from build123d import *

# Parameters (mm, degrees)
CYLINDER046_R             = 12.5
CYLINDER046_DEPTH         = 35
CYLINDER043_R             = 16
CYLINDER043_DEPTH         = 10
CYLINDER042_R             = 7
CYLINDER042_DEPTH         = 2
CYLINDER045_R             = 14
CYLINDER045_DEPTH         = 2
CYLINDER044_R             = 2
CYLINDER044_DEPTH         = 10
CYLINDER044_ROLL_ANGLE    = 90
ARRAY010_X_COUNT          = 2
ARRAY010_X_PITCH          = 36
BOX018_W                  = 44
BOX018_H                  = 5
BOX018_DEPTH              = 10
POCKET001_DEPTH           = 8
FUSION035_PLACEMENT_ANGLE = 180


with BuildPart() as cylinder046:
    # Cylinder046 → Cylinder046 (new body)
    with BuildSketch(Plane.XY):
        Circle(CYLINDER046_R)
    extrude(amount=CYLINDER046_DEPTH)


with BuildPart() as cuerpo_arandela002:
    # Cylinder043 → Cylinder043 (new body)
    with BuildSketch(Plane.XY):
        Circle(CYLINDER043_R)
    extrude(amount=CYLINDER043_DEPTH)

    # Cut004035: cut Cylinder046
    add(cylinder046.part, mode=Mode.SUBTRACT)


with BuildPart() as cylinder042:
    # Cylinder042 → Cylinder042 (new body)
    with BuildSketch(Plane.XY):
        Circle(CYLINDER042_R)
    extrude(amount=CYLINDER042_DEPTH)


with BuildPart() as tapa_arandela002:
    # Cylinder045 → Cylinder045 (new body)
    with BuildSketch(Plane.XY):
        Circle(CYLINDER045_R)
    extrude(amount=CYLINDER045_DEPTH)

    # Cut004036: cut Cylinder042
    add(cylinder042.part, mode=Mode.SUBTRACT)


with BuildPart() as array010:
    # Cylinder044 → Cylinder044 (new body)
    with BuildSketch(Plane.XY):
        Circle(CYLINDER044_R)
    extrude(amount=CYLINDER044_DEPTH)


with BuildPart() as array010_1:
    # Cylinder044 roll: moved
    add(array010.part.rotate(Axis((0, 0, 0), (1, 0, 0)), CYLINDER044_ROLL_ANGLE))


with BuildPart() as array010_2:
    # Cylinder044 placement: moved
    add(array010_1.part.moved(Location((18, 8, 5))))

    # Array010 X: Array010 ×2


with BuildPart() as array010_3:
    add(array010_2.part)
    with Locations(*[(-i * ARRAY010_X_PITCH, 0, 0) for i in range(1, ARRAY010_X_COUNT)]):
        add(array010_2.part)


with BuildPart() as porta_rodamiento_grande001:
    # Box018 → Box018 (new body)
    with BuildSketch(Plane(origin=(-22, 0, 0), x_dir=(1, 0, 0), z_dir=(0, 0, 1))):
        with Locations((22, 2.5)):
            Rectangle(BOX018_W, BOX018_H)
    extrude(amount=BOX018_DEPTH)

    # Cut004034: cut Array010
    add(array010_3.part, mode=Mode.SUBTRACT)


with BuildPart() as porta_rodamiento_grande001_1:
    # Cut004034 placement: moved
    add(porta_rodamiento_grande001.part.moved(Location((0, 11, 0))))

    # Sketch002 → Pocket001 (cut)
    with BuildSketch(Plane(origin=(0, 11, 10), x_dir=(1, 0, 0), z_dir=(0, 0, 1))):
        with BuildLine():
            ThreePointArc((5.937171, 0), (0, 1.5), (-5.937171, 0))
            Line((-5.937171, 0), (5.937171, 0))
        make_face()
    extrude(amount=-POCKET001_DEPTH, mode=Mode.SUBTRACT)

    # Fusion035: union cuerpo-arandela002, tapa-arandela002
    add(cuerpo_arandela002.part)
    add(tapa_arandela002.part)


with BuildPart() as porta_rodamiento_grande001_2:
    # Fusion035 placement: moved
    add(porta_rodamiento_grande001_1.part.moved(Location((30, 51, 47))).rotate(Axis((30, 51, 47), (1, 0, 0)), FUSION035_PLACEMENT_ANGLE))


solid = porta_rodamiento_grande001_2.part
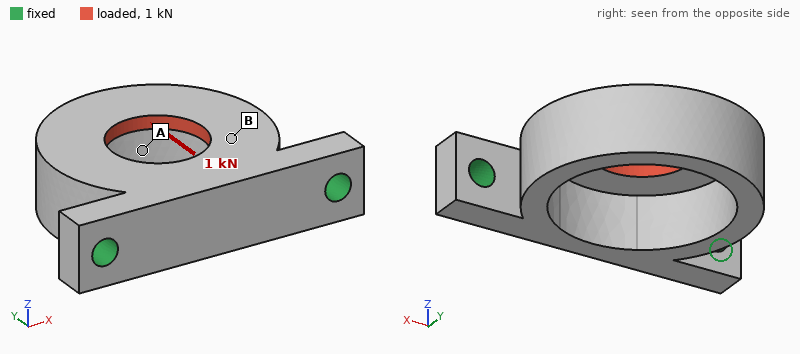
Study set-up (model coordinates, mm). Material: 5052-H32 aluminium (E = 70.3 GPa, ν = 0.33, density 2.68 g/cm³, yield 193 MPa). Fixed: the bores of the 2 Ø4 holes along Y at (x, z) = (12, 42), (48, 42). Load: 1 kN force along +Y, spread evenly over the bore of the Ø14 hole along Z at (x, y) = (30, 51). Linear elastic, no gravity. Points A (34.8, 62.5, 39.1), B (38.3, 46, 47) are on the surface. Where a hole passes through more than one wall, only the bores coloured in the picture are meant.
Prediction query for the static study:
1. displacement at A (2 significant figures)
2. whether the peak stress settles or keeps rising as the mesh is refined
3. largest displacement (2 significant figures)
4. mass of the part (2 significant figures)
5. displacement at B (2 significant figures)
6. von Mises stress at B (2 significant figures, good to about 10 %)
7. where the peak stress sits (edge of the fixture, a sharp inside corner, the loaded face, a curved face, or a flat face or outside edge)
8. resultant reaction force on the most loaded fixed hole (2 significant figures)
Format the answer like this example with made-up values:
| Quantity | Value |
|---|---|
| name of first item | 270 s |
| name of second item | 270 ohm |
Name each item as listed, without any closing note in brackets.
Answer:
| Quantity | Value |
|---|---|
| displacement at A | 49 µm |
| whether the peak stress settles or keeps rising as the mesh is refined | keeps rising |
| largest displacement | 64 µm |
| mass of the part | 14 g |
| displacement at B | 23 µm |
| von Mises stress at B | 27 MPa |
| where the peak stress sits | edge of the fixture |
| resultant reaction force on the most loaded fixed hole | 510 N |
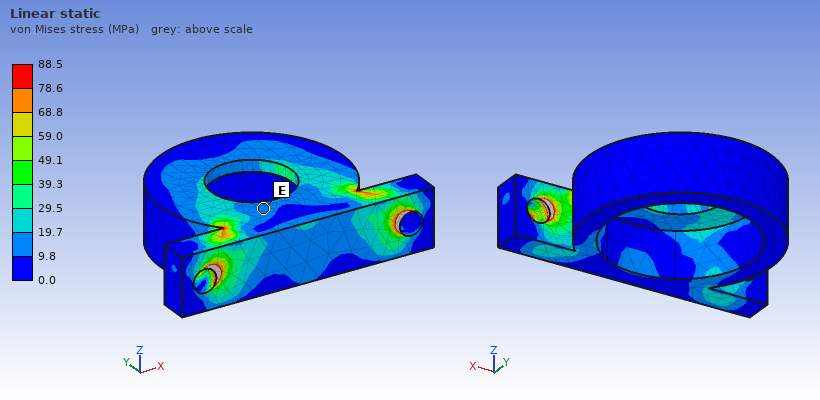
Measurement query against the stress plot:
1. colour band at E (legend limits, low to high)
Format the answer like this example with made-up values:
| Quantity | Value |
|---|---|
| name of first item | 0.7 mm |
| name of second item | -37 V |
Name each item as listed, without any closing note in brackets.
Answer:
| Quantity | Value |
|---|---|
| colour band at E | 9.8 to 19.7 MPa |
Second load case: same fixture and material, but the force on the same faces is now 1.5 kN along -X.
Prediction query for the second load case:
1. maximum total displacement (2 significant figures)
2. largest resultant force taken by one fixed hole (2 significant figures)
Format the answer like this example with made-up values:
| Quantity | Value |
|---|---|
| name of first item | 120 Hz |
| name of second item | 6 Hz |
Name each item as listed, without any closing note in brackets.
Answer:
| Quantity | Value |
|---|---|
| maximum total displacement | 75 µm |
| largest resultant force taken by one fixed hole | 1.0 kN |
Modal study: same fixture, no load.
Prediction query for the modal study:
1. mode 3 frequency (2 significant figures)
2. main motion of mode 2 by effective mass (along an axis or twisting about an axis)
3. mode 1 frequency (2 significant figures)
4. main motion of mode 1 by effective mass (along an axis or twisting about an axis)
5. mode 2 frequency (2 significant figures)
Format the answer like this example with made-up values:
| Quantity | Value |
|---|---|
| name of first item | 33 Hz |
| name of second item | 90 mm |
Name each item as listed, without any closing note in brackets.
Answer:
| Quantity | Value |
|---|---|
| mode 3 frequency | 12 kHz |
| main motion of mode 2 by effective mass | along X |
| mode 1 frequency | 3900 Hz |
| main motion of mode 1 by effective mass | along Z |
| mode 2 frequency | 7000 Hz |
